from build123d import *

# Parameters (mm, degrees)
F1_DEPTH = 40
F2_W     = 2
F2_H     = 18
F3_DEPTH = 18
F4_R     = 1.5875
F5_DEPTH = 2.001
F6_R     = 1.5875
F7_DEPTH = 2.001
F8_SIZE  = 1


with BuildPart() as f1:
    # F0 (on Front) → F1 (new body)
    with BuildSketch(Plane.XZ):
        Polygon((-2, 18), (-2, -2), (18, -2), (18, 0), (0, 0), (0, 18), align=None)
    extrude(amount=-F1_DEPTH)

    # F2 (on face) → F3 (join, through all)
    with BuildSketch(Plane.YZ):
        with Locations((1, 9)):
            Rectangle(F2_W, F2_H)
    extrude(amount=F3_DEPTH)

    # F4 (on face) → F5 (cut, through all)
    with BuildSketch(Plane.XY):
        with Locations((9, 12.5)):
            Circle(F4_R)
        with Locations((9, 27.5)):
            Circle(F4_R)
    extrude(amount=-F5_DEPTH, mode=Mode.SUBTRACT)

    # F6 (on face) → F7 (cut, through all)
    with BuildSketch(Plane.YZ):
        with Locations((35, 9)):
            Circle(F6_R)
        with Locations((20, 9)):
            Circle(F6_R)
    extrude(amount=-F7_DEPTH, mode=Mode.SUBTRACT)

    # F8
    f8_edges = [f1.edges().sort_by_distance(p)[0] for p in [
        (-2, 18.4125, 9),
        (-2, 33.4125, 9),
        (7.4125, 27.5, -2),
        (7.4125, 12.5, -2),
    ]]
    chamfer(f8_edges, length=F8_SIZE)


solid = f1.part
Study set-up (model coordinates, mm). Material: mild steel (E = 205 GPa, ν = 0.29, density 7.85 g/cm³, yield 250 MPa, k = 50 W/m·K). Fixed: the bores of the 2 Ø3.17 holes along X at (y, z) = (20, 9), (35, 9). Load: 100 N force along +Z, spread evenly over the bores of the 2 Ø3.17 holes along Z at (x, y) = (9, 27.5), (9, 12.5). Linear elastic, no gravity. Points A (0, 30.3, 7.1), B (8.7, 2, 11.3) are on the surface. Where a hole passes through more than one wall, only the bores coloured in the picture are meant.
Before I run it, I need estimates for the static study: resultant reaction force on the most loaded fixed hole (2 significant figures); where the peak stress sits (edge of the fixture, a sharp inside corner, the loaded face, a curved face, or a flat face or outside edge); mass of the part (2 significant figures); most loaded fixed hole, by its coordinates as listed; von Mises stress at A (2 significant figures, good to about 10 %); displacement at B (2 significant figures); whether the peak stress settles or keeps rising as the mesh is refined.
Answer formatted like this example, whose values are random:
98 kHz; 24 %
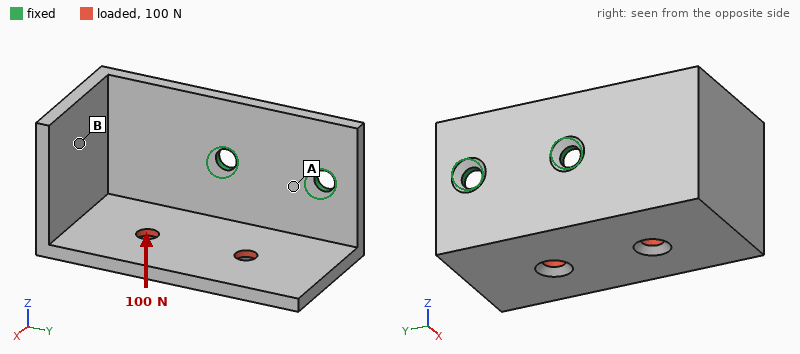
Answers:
99 N; edge of the fixture; 28 g; (20, 9); 30 MPa; 22 µm; keeps rising
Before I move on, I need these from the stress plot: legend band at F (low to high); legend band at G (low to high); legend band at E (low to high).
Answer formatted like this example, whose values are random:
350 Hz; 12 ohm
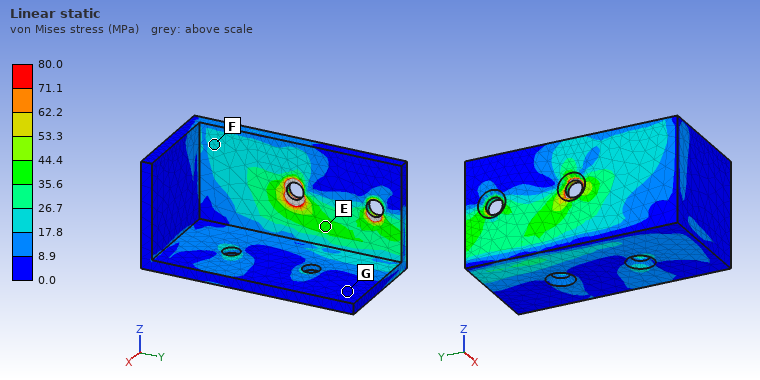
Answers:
17.8 to 26.7 MPa; 0.0 to 8.9 MPa; 35.6 to 44.4 MPa
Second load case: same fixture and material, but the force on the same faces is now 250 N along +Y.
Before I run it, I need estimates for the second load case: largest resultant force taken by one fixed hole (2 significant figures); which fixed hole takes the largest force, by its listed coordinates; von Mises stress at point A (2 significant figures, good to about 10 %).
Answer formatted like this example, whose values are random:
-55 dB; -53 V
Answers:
250 N; (20, 9); 41 MPa
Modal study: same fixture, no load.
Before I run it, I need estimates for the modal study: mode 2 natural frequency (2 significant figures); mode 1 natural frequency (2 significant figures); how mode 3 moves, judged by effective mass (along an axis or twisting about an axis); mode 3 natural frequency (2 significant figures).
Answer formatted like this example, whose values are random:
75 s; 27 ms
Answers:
2500 Hz; 1900 Hz; along X; 4000 Hz
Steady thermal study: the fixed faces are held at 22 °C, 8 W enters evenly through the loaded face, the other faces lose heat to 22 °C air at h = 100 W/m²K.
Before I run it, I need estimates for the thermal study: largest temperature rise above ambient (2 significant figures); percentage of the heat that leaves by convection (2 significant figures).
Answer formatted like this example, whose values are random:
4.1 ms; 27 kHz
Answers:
34 K; 60 %
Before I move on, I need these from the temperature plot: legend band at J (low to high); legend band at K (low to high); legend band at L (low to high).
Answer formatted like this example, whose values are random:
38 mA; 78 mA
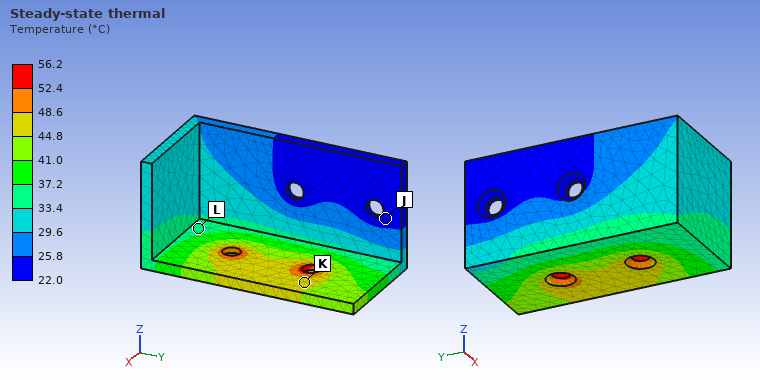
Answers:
22.0 to 25.8 °C; 44.8 to 48.6 °C; 33.4 to 37.2 °C
